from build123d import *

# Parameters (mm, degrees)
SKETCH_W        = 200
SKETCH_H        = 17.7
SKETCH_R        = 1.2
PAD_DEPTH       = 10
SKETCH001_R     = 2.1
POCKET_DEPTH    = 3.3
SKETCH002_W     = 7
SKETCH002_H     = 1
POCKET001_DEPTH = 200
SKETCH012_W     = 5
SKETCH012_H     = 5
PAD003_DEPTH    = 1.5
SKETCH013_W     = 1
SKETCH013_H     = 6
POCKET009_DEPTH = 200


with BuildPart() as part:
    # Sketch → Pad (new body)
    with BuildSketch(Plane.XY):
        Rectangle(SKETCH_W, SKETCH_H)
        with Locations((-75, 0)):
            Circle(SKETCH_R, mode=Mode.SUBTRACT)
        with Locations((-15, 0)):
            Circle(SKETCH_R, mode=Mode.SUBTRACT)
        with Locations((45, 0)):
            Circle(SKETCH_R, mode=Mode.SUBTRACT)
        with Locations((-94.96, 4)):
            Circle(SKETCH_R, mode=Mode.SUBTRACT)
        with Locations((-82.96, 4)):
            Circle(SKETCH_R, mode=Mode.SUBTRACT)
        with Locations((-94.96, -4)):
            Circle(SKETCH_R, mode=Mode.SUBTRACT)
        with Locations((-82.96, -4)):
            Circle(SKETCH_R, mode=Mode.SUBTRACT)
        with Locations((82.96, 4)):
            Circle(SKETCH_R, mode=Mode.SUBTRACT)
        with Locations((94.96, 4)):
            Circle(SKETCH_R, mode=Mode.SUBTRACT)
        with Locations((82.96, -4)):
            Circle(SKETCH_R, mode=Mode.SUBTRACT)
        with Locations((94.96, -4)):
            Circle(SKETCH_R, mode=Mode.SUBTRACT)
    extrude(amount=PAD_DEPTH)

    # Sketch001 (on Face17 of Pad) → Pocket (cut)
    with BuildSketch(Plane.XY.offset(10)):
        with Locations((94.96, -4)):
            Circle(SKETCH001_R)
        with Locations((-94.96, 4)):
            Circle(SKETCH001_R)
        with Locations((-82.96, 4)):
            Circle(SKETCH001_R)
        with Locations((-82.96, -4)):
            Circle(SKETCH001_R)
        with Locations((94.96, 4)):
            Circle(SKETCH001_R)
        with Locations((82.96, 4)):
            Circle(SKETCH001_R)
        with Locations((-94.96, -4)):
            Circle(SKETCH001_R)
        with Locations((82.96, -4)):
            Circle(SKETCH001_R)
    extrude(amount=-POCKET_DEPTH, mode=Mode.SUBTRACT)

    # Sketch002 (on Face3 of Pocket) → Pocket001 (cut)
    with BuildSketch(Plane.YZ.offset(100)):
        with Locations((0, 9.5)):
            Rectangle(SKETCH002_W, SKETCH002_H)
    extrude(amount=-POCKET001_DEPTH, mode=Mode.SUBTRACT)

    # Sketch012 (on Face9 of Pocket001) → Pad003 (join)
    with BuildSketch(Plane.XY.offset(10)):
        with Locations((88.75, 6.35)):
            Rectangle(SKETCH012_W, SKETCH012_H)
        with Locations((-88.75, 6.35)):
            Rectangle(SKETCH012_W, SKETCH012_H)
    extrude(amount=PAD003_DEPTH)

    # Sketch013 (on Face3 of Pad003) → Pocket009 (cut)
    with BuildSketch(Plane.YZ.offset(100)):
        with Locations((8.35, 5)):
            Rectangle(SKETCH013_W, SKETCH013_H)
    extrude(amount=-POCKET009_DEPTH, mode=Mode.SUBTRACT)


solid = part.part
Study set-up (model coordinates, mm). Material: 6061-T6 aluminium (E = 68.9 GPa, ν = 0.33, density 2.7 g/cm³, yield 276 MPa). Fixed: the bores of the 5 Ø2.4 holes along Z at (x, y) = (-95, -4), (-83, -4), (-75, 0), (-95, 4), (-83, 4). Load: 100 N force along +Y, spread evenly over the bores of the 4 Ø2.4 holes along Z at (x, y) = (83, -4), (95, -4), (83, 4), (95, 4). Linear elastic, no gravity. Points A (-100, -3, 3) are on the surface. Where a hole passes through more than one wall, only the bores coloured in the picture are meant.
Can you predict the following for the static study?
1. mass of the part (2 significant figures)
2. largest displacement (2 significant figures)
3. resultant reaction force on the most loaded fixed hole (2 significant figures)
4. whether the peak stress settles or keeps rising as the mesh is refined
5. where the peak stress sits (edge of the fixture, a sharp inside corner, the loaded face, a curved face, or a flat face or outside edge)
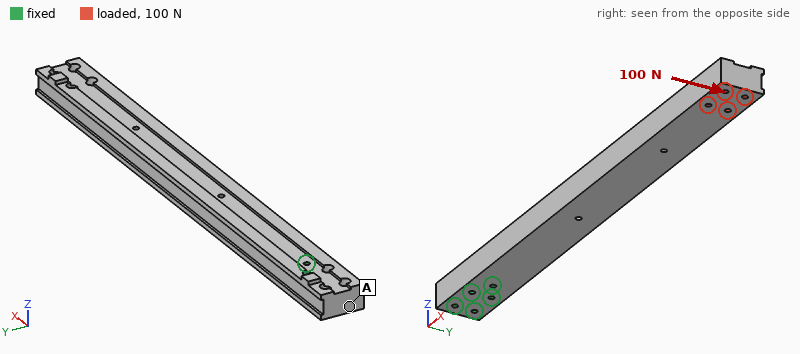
87 g
0.65 mm
810 N
keeps rising
edge of the fixture
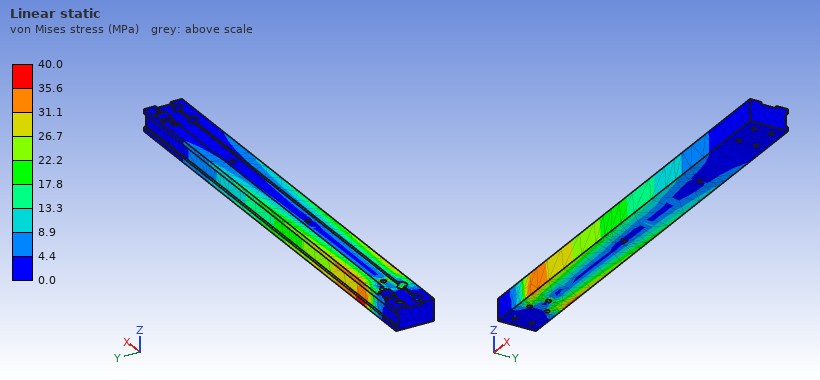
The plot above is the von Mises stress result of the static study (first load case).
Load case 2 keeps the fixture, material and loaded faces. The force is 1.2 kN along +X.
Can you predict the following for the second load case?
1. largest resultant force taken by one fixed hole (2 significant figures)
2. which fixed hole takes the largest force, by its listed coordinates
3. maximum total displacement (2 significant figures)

750 N
(-75, 0)
0.30 mm
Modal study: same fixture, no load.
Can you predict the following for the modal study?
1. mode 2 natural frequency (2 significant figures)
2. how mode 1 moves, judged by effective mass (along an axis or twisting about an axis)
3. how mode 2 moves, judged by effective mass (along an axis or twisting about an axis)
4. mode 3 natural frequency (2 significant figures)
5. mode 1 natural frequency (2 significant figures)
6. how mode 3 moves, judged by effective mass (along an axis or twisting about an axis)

430 Hz
along Z
along Y
1600 Hz
260 Hz
along Z
